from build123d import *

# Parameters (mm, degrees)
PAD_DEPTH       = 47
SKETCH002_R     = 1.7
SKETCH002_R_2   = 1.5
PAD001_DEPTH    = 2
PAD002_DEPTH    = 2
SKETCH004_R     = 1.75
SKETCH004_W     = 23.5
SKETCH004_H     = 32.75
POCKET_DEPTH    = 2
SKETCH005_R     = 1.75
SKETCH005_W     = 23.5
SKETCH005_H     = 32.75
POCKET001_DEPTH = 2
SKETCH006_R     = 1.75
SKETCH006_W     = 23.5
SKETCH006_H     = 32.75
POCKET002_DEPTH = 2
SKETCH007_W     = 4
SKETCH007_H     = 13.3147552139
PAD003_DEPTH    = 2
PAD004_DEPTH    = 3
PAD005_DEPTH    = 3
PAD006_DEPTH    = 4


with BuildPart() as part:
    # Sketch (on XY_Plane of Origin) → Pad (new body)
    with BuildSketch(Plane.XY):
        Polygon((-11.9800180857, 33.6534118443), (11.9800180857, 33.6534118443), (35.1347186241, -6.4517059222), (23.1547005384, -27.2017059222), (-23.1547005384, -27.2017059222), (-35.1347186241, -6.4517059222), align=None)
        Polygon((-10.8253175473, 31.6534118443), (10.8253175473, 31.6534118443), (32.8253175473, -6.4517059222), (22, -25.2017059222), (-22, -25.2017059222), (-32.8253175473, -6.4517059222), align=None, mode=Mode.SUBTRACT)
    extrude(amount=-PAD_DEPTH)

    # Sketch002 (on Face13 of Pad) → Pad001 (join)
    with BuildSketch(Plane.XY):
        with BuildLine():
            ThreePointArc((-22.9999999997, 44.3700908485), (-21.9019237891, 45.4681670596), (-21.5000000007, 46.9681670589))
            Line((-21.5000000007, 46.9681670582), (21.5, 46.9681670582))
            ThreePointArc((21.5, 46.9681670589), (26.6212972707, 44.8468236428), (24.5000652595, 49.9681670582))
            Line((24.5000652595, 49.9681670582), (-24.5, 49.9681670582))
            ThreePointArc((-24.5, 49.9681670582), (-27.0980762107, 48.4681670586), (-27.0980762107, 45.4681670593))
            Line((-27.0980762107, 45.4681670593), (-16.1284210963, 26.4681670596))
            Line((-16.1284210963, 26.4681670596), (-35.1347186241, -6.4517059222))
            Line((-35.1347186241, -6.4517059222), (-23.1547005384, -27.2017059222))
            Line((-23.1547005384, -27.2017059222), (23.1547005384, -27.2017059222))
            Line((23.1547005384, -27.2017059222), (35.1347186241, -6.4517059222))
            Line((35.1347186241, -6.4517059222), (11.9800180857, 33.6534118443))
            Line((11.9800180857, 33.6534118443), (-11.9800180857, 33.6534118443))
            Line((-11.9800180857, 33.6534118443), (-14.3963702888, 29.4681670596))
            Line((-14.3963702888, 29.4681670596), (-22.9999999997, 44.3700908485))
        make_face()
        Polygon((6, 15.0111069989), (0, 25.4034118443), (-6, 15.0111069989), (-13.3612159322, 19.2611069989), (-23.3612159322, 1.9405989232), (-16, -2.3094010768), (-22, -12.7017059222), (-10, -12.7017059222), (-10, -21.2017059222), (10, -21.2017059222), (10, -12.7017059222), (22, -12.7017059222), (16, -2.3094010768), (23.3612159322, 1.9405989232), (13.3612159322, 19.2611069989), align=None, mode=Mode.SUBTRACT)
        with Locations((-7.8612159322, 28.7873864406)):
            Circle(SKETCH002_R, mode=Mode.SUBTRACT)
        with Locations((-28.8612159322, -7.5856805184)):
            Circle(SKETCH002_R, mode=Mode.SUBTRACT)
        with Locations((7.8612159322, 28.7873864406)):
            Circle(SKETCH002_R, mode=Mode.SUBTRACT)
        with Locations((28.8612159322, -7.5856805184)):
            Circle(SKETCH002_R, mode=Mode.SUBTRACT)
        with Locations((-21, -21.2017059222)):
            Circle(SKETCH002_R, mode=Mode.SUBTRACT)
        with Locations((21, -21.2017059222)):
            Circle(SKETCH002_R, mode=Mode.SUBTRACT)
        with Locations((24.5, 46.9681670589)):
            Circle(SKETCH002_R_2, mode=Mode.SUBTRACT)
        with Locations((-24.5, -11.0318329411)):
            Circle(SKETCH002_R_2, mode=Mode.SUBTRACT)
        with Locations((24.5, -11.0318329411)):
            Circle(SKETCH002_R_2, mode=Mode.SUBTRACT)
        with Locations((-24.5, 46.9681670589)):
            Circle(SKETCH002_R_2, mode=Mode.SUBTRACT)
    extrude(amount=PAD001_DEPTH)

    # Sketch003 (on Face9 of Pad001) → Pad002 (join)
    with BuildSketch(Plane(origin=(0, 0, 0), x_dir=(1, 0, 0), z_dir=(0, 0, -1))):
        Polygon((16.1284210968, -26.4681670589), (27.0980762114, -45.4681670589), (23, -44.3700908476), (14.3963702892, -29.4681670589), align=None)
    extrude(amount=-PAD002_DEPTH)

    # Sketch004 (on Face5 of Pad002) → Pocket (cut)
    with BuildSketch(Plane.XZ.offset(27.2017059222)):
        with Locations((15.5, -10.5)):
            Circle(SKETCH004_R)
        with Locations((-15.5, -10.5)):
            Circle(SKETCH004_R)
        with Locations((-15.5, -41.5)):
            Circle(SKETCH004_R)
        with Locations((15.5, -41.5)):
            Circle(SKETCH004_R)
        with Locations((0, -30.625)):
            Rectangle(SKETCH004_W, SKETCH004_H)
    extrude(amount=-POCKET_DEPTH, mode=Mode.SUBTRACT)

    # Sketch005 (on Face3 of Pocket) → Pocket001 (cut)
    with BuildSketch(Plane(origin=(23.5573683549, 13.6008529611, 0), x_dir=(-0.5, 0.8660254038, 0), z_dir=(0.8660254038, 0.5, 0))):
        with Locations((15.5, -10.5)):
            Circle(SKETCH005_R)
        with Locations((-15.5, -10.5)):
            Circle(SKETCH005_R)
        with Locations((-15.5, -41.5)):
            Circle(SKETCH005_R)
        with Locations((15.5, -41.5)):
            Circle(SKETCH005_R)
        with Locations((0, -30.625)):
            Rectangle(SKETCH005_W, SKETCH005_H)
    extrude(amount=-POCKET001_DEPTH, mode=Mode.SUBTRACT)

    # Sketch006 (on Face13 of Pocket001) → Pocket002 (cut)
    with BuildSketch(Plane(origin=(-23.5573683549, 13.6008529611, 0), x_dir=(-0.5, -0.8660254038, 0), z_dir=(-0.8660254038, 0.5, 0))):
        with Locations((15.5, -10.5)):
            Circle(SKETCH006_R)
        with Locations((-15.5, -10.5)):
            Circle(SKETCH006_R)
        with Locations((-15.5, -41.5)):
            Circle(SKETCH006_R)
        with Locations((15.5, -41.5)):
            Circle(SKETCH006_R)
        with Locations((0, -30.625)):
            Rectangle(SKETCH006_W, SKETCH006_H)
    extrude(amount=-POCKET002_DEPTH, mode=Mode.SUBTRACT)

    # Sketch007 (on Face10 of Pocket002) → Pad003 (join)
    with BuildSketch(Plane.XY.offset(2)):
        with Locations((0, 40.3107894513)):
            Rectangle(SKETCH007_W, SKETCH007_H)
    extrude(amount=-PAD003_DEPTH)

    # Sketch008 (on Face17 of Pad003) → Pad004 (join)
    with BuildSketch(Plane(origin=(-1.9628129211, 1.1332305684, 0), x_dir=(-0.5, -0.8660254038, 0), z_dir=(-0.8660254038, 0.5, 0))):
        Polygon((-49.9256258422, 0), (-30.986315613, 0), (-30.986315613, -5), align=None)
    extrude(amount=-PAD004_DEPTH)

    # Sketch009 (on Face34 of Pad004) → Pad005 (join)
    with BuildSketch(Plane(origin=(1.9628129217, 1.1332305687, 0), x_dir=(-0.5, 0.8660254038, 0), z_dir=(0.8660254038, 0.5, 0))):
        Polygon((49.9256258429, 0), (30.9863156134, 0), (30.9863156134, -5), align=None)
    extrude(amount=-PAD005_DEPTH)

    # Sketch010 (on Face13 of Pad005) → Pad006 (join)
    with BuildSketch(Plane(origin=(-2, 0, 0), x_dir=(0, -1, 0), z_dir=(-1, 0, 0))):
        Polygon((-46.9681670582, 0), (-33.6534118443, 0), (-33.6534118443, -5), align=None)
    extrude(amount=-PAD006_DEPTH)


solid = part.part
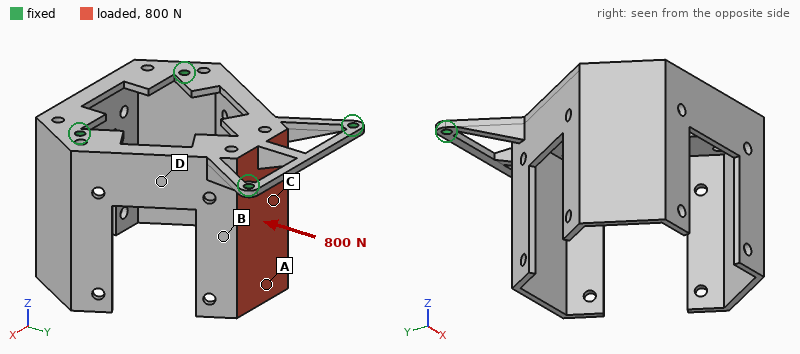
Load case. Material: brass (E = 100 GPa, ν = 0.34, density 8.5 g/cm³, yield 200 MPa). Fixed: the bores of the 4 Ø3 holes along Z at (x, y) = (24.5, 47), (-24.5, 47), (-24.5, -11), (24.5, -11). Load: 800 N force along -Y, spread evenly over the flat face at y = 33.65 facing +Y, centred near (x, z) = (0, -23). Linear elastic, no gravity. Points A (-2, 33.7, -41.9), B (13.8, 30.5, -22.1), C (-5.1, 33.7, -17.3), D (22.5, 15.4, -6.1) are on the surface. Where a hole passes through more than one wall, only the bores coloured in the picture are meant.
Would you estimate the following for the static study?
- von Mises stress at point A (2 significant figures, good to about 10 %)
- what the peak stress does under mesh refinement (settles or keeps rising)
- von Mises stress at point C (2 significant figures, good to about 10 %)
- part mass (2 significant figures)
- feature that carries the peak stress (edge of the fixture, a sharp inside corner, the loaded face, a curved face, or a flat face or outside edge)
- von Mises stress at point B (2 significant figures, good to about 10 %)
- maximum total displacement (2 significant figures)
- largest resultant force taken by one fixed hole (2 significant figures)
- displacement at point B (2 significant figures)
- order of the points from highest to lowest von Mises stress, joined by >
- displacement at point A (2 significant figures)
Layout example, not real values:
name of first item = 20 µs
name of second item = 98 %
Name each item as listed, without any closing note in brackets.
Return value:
von Mises stress at point A = 66 MPa
what the peak stress does under mesh refinement = keeps rising
von Mises stress at point C = 45 MPa
part mass = 160 g
feature that carries the peak stress = edge of the fixture
von Mises stress at point B = 23 MPa
maximum total displacement = 0.31 mm
largest resultant force taken by one fixed hole = 330 N
displacement at point B = 0.12 mm
order of the points from highest to lowest von Mises stress, joined by > = A > C > B > D
displacement at point A = 0.27 mm
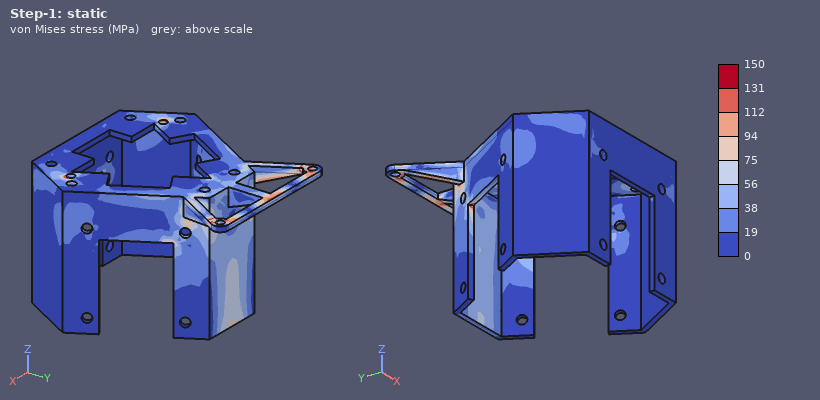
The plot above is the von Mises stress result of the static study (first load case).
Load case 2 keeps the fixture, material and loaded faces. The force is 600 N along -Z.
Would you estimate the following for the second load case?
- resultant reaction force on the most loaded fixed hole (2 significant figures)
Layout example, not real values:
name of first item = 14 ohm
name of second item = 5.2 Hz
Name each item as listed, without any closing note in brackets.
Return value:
resultant reaction force on the most loaded fixed hole = 340 N
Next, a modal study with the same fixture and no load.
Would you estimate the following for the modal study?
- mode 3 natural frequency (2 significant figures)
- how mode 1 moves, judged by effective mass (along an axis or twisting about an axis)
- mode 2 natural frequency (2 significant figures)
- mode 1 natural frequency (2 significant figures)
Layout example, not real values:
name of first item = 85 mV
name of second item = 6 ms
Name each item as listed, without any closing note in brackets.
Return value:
mode 3 natural frequency = 1300 Hz
how mode 1 moves, judged by effective mass = along Y
mode 2 natural frequency = 1000 Hz
mode 1 natural frequency = 780 Hz
